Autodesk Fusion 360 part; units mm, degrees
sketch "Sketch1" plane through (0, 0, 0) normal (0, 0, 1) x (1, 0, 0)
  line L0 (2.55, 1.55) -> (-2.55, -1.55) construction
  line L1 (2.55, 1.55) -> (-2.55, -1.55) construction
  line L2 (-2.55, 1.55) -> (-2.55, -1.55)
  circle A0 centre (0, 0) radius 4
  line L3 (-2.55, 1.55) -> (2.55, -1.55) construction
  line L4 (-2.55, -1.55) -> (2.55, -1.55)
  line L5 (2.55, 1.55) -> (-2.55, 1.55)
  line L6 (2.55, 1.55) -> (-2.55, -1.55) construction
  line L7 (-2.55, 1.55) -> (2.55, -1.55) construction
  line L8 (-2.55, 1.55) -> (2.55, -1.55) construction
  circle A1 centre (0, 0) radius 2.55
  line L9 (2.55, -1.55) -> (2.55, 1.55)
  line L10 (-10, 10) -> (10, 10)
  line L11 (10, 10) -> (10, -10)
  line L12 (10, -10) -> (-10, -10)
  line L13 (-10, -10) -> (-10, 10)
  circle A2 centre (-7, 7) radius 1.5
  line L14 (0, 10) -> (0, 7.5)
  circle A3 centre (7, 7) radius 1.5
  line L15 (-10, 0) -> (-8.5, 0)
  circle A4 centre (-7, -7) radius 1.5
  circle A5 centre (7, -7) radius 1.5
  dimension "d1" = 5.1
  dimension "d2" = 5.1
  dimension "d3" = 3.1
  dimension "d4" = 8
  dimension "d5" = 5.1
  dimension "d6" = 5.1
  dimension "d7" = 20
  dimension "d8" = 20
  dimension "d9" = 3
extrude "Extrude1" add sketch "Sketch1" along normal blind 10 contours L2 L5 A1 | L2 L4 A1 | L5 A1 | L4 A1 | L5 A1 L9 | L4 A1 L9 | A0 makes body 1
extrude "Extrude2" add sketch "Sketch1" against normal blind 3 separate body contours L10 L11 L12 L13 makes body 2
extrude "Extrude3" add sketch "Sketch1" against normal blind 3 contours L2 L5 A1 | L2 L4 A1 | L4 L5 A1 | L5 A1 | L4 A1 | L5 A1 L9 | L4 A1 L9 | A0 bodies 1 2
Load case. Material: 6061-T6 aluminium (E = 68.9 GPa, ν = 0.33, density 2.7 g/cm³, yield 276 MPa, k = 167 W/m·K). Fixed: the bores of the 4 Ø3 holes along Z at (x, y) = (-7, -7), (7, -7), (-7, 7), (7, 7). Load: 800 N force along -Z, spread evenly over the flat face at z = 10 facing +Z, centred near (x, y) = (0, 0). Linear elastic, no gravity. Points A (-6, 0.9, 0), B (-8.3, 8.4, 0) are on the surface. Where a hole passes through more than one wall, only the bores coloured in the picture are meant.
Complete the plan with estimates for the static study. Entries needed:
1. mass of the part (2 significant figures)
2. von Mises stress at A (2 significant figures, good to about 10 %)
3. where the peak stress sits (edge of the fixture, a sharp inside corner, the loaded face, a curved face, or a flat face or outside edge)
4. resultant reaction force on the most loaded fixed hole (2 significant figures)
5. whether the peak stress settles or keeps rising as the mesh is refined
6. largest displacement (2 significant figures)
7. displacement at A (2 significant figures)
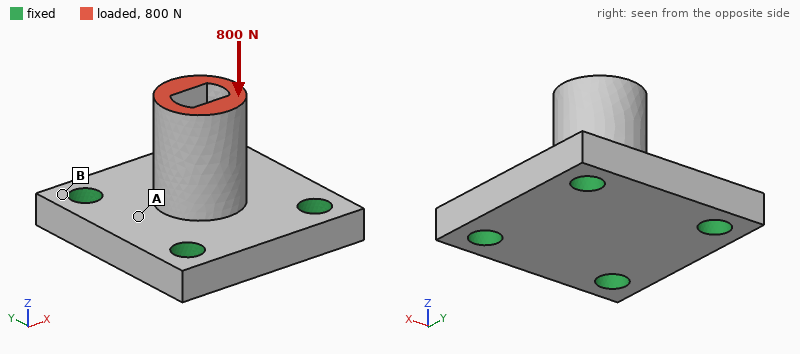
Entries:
4.0 g
17 MPa
edge of the fixture
200 N
keeps rising
9.1 µm
3.4 µm
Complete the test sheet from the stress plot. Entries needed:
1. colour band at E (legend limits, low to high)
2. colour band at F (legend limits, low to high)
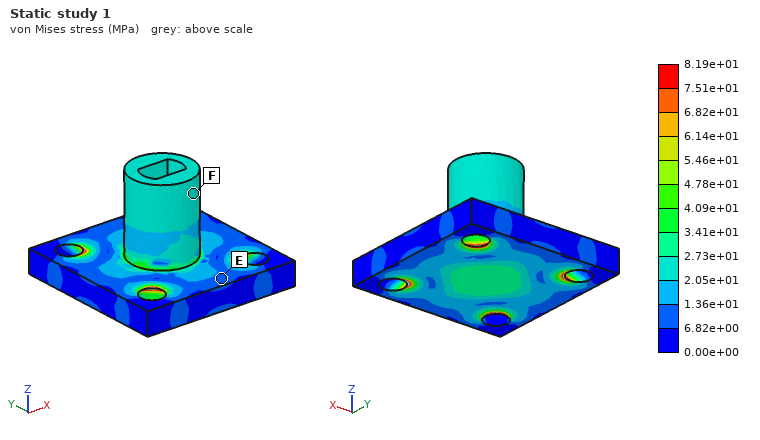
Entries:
6.82e+00 to 1.36e+01 MPa
2.05e+01 to 2.73e+01 MPa
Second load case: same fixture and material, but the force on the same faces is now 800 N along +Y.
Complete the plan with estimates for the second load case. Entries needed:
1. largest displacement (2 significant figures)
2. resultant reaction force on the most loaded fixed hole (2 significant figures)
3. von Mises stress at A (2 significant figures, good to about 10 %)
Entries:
78 µm
460 N
45 MPa
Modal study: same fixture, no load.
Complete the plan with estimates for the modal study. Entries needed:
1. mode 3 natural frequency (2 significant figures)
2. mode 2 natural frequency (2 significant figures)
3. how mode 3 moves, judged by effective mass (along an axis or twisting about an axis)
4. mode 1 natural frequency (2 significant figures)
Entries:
42 kHz
29 kHz
along Z
28 kHz
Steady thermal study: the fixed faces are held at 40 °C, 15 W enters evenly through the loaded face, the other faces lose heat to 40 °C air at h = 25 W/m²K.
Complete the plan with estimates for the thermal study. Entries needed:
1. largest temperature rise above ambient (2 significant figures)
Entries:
32 K
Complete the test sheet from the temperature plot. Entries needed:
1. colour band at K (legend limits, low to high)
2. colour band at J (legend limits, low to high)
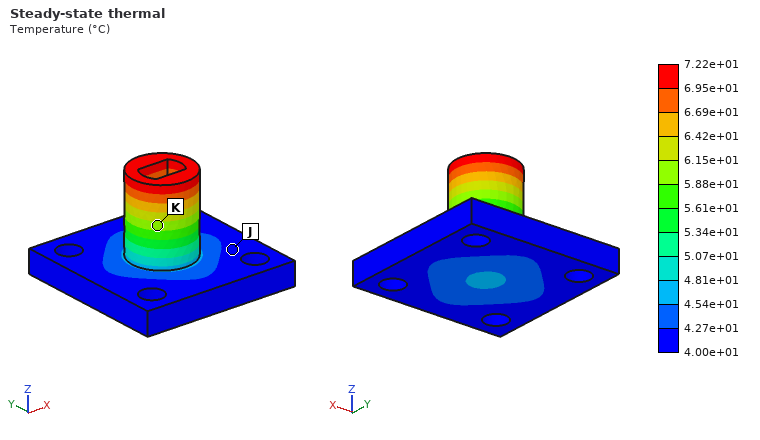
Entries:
5.88e+01 to 6.15e+01 °C
4.00e+01 to 4.27e+01 °C
